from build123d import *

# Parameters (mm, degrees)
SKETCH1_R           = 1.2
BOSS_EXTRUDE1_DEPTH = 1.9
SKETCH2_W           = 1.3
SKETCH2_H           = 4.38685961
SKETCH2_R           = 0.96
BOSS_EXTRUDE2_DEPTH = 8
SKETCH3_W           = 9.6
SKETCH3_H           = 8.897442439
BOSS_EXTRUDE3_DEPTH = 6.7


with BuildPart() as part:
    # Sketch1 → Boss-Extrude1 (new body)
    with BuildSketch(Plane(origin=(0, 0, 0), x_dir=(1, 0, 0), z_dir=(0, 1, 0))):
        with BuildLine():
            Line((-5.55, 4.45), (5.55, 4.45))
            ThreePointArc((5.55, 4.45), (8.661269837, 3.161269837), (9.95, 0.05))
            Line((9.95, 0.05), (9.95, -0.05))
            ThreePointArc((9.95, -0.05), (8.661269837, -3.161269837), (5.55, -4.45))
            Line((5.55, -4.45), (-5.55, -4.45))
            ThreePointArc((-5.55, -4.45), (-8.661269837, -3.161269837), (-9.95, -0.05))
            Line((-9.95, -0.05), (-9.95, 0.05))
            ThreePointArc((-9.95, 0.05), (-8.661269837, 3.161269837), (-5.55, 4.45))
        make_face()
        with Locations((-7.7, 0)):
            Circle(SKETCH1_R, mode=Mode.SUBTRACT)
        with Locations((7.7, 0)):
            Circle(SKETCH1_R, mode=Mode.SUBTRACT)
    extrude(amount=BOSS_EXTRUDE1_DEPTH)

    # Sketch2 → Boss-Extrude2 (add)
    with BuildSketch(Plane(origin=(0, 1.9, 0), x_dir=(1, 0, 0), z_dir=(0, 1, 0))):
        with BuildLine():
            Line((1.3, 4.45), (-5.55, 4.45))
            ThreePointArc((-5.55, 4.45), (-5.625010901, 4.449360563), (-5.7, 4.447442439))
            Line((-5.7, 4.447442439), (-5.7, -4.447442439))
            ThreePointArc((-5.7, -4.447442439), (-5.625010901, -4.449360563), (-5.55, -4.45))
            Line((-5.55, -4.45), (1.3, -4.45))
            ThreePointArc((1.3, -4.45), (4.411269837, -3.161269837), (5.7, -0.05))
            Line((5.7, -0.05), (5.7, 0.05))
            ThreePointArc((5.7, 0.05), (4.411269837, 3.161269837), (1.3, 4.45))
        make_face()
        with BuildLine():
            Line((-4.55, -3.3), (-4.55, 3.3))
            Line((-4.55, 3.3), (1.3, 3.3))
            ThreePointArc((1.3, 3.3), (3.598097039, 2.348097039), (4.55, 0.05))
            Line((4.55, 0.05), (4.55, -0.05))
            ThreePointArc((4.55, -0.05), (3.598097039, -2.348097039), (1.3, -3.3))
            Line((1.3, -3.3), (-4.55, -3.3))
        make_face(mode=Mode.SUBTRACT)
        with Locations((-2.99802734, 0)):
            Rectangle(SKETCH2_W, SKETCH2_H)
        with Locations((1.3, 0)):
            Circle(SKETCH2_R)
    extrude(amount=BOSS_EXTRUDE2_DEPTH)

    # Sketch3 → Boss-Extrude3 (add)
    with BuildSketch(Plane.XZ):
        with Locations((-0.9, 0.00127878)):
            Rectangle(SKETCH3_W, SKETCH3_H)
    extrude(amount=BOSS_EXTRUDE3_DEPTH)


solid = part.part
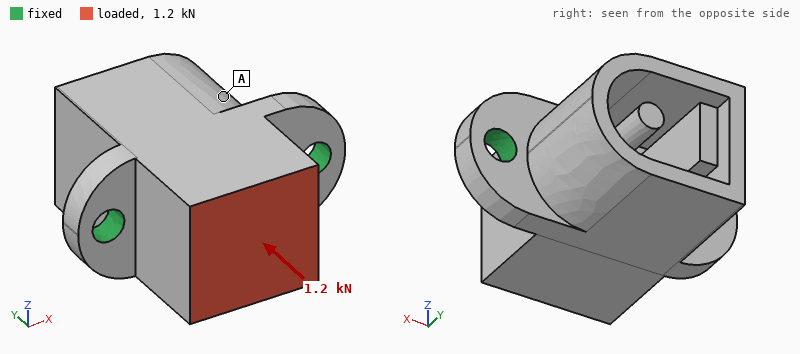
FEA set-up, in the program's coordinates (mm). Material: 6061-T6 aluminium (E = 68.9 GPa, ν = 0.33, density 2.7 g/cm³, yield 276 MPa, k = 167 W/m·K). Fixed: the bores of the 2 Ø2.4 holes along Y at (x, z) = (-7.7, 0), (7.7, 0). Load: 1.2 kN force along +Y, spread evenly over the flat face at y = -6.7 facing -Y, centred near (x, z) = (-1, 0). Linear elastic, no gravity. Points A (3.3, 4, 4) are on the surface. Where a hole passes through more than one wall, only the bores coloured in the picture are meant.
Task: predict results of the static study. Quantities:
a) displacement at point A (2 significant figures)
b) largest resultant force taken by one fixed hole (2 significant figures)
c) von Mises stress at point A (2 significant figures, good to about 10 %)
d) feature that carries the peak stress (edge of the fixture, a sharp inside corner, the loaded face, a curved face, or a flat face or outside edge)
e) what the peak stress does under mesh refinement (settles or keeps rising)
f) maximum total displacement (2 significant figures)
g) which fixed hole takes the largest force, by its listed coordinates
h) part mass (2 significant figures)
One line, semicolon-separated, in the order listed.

10 µm; 680 N; 31 MPa; edge of the fixture; keeps rising; 14 µm; (-7.7, 0); 3.3 g
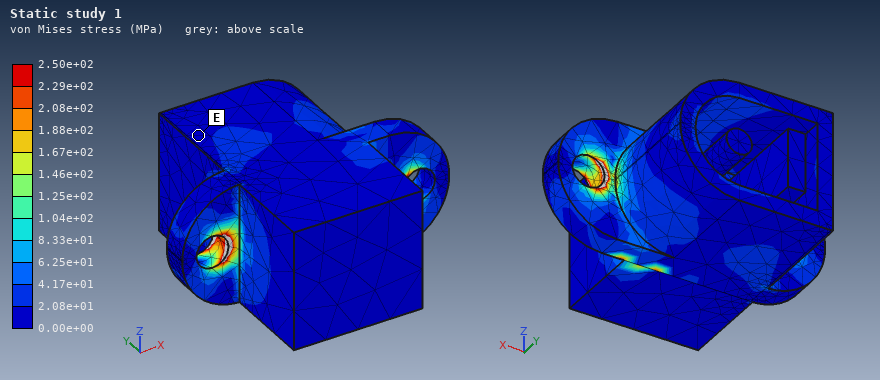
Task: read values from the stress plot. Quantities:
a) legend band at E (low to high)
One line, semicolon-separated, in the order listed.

0.00e+00 to 2.08e+01 MPa
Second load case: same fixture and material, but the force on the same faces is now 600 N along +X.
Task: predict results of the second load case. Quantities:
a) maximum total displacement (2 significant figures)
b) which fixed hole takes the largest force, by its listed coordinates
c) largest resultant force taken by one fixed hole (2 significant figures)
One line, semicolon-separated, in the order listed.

15 µm; (-7.7, 0); 520 N
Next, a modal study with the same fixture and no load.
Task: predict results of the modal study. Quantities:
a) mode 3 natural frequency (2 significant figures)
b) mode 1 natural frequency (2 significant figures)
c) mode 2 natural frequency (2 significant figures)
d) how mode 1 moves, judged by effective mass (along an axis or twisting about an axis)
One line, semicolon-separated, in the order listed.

19 kHz; 12 kHz; 15 kHz; twisting about X
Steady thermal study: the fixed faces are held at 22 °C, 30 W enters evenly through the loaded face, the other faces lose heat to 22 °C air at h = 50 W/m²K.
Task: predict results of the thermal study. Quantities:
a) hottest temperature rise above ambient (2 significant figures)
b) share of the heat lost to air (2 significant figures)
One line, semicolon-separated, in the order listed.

34 K; 3.5 %
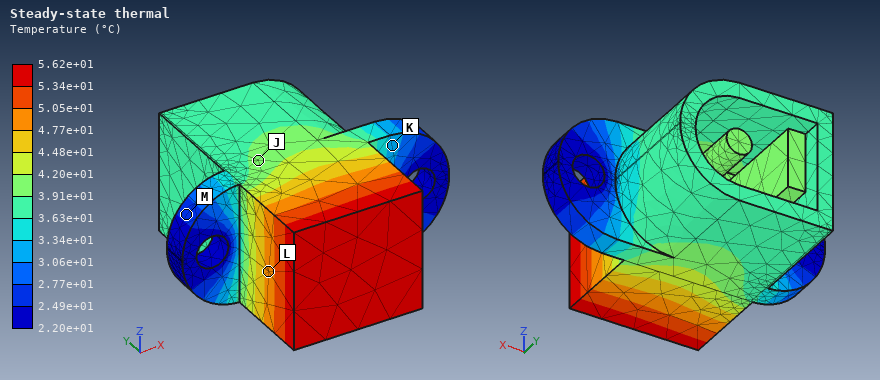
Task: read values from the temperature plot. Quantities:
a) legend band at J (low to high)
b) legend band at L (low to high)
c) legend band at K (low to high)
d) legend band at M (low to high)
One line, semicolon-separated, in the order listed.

3.91e+01 to 4.20e+01 °C; 4.77e+01 to 5.05e+01 °C; 3.06e+01 to 3.34e+01 °C; 2.49e+01 to 2.77e+01 °C
